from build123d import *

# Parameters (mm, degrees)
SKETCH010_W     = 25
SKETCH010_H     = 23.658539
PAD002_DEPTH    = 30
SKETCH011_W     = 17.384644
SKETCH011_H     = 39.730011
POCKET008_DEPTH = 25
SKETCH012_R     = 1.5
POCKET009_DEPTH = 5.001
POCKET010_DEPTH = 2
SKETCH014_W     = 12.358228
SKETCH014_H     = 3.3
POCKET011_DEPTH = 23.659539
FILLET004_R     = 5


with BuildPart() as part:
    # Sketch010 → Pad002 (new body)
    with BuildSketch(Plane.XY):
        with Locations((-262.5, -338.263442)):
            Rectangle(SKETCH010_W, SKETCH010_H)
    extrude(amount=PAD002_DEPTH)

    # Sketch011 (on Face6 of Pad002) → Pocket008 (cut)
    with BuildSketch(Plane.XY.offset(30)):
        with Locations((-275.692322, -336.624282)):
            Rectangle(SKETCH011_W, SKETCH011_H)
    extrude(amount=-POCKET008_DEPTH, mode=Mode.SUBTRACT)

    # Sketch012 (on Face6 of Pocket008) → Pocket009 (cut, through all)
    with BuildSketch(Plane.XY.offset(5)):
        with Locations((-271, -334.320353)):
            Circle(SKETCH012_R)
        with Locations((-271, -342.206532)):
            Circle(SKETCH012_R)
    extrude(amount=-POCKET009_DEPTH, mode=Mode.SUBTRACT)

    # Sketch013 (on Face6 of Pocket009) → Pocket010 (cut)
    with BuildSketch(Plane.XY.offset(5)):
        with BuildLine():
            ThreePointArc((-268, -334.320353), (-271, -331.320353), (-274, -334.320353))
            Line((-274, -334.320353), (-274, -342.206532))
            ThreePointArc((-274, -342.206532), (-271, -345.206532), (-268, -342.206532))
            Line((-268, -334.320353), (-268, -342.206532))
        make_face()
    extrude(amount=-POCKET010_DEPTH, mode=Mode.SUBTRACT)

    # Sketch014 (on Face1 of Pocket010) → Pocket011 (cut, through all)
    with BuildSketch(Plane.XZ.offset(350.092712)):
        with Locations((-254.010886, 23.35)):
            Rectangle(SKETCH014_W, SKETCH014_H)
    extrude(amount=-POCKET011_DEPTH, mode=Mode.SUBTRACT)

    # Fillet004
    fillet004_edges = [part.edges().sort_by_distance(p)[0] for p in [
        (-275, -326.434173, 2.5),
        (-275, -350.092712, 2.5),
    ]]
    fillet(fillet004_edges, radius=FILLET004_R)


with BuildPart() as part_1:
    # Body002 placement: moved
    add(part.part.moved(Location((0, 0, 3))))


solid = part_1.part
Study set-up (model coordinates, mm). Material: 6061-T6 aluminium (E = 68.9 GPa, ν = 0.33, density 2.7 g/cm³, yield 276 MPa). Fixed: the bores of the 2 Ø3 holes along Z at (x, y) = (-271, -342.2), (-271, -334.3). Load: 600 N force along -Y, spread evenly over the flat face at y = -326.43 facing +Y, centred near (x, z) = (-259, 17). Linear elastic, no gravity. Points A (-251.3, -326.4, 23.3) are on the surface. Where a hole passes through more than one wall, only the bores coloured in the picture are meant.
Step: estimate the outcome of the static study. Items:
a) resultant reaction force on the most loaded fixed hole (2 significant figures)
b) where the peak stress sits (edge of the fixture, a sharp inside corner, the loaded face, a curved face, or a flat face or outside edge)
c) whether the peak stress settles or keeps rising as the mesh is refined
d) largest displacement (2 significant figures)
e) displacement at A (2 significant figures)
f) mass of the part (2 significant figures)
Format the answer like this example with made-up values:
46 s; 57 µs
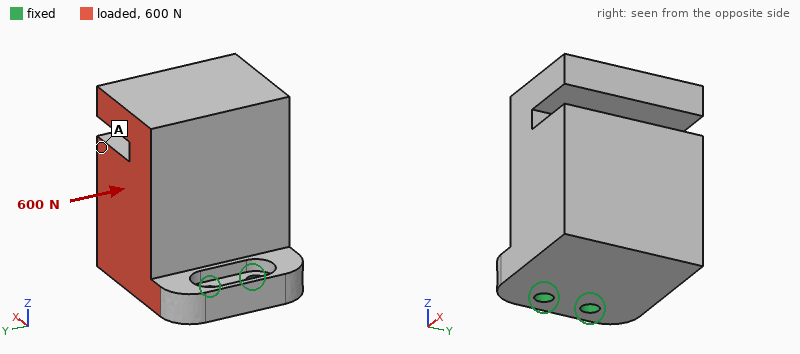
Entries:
970 N; edge of the fixture; keeps rising; 52 µm; 38 µm; 32 g
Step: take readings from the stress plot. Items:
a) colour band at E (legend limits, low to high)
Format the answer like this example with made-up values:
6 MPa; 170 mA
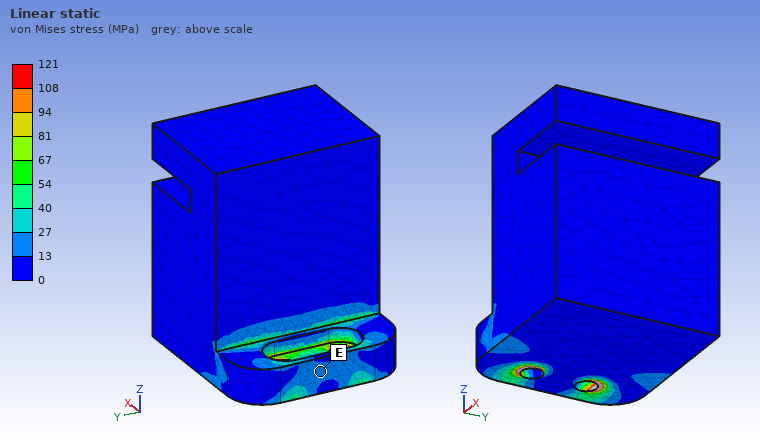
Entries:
13 to 27 MPa
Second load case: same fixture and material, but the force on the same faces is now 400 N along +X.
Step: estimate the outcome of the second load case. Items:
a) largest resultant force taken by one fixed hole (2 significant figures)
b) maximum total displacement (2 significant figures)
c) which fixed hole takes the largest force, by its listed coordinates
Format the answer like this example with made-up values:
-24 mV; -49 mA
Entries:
650 N; 0.15 mm; (-271, -334.3)
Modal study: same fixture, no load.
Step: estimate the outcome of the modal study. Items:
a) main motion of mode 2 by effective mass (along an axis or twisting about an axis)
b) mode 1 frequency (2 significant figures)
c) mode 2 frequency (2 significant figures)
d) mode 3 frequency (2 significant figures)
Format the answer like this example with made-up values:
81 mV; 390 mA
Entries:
along Y; 1600 Hz; 3700 Hz; 8500 Hz
